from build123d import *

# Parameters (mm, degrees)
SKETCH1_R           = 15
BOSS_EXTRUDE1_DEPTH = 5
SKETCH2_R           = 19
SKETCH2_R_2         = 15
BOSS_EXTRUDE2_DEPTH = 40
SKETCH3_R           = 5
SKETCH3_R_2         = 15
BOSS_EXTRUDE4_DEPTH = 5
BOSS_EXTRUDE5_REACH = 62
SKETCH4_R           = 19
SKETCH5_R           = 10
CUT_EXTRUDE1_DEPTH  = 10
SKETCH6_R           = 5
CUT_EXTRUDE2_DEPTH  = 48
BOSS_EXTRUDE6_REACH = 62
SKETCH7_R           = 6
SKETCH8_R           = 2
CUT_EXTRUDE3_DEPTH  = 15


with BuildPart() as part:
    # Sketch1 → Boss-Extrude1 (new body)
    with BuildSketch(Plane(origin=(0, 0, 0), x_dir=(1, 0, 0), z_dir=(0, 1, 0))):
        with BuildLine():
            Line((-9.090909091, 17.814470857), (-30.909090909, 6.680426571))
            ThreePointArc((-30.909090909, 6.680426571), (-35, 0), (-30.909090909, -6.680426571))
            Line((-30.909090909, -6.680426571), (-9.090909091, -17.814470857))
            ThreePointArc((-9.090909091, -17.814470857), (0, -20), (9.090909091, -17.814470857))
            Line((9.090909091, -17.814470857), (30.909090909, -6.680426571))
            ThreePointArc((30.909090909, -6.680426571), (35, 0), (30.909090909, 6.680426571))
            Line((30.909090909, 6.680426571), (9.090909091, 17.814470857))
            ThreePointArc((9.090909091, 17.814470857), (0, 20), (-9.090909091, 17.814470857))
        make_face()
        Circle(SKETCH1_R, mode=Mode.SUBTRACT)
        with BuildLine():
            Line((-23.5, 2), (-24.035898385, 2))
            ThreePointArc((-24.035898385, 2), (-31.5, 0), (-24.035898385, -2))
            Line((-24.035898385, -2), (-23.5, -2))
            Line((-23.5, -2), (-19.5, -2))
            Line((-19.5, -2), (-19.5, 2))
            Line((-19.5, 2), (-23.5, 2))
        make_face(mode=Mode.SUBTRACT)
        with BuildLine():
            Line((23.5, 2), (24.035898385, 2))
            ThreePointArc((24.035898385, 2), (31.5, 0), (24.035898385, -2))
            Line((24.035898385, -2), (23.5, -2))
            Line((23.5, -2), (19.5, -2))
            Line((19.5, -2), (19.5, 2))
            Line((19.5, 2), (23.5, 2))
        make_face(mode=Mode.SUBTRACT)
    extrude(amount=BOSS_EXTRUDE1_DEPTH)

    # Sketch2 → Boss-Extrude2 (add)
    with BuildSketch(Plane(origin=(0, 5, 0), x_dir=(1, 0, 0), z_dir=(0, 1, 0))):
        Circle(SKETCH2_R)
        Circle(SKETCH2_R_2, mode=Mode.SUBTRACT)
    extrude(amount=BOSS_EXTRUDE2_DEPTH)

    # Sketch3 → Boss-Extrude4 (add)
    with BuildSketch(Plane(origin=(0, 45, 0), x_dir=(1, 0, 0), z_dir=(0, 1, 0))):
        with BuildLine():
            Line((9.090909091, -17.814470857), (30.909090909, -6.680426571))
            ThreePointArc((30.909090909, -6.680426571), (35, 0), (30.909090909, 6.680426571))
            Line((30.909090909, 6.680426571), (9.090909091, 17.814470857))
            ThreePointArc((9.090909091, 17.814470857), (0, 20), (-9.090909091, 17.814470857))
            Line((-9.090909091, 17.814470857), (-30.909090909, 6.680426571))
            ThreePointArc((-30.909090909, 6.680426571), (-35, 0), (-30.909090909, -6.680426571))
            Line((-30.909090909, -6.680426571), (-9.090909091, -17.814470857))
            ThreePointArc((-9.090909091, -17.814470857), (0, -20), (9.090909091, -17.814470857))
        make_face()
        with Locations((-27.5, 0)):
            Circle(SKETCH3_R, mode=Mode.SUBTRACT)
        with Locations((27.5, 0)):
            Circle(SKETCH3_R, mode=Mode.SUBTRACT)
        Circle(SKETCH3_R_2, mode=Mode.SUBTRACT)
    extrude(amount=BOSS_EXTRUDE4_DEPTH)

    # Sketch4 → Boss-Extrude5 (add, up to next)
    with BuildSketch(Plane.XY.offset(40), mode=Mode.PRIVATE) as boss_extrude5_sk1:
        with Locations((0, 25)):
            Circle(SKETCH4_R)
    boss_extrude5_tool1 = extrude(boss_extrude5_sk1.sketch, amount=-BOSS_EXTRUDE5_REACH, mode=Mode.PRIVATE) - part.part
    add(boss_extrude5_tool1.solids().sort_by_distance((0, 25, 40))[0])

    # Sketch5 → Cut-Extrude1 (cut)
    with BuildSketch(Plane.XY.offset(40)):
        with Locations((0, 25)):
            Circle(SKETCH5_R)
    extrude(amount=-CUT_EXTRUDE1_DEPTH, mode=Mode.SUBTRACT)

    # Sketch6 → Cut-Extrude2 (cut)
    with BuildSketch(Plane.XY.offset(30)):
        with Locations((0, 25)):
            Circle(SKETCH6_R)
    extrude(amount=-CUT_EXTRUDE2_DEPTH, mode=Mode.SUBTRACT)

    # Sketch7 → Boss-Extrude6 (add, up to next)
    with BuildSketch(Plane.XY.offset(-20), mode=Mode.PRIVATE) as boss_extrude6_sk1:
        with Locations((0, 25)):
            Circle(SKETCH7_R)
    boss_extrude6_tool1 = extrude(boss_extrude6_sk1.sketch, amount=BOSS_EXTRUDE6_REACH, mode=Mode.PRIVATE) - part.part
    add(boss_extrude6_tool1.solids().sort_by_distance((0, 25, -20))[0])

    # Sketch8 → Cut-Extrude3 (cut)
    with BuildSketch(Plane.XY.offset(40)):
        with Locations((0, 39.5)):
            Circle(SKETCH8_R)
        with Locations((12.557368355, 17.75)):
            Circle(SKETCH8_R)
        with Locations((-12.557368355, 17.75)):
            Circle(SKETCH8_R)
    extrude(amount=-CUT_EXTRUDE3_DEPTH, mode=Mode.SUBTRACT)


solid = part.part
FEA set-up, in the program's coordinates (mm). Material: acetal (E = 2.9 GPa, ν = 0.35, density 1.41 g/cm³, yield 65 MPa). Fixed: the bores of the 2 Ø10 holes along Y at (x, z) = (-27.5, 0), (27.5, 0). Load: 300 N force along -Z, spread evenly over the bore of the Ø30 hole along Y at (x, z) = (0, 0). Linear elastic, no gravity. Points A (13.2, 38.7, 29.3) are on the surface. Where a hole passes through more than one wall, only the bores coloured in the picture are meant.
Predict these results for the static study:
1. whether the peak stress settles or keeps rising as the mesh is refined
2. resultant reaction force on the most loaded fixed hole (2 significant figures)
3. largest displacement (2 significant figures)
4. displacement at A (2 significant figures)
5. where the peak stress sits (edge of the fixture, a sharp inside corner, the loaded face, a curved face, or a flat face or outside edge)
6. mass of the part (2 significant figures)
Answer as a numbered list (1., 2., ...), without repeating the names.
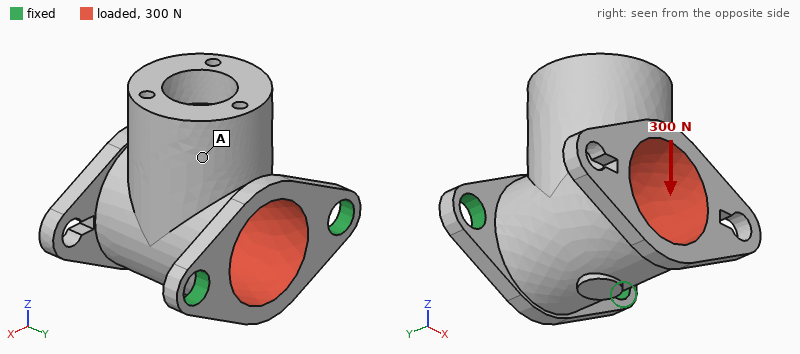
1. keeps rising
2. 150 N
3. 1.2 mm
4. 0.62 mm
5. edge of the fixture
6. 69 g
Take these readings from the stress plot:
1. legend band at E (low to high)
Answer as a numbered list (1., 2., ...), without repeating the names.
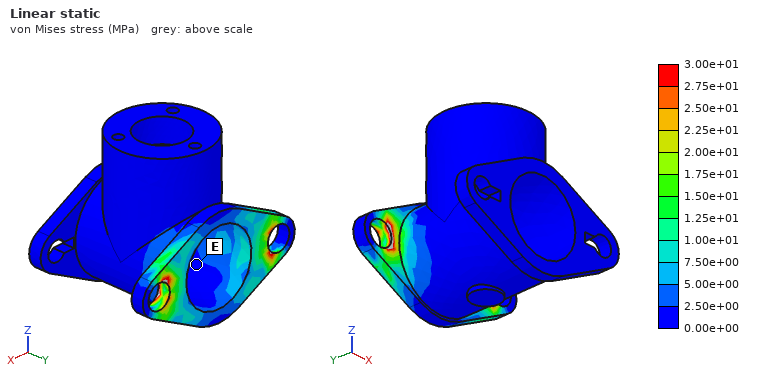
1. 0.00e+00 to 2.50e+00 MPa
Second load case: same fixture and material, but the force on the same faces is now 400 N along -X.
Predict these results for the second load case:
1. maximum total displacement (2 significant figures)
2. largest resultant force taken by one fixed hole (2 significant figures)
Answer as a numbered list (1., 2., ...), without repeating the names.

1. 0.16 mm
2. 300 N
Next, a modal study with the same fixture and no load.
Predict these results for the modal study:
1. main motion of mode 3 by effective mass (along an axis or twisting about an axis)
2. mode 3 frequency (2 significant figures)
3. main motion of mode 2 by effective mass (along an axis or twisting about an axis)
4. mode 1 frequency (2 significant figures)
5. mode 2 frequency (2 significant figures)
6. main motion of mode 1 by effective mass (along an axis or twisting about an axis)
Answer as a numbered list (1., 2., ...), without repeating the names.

1. along Y
2. 1800 Hz
3. along X
4. 330 Hz
5. 1100 Hz
6. along Z
